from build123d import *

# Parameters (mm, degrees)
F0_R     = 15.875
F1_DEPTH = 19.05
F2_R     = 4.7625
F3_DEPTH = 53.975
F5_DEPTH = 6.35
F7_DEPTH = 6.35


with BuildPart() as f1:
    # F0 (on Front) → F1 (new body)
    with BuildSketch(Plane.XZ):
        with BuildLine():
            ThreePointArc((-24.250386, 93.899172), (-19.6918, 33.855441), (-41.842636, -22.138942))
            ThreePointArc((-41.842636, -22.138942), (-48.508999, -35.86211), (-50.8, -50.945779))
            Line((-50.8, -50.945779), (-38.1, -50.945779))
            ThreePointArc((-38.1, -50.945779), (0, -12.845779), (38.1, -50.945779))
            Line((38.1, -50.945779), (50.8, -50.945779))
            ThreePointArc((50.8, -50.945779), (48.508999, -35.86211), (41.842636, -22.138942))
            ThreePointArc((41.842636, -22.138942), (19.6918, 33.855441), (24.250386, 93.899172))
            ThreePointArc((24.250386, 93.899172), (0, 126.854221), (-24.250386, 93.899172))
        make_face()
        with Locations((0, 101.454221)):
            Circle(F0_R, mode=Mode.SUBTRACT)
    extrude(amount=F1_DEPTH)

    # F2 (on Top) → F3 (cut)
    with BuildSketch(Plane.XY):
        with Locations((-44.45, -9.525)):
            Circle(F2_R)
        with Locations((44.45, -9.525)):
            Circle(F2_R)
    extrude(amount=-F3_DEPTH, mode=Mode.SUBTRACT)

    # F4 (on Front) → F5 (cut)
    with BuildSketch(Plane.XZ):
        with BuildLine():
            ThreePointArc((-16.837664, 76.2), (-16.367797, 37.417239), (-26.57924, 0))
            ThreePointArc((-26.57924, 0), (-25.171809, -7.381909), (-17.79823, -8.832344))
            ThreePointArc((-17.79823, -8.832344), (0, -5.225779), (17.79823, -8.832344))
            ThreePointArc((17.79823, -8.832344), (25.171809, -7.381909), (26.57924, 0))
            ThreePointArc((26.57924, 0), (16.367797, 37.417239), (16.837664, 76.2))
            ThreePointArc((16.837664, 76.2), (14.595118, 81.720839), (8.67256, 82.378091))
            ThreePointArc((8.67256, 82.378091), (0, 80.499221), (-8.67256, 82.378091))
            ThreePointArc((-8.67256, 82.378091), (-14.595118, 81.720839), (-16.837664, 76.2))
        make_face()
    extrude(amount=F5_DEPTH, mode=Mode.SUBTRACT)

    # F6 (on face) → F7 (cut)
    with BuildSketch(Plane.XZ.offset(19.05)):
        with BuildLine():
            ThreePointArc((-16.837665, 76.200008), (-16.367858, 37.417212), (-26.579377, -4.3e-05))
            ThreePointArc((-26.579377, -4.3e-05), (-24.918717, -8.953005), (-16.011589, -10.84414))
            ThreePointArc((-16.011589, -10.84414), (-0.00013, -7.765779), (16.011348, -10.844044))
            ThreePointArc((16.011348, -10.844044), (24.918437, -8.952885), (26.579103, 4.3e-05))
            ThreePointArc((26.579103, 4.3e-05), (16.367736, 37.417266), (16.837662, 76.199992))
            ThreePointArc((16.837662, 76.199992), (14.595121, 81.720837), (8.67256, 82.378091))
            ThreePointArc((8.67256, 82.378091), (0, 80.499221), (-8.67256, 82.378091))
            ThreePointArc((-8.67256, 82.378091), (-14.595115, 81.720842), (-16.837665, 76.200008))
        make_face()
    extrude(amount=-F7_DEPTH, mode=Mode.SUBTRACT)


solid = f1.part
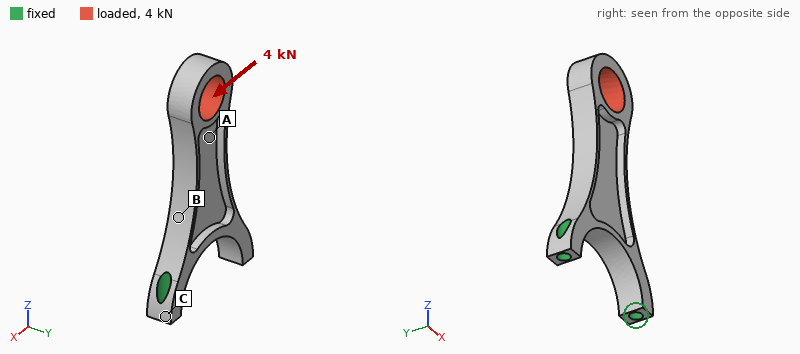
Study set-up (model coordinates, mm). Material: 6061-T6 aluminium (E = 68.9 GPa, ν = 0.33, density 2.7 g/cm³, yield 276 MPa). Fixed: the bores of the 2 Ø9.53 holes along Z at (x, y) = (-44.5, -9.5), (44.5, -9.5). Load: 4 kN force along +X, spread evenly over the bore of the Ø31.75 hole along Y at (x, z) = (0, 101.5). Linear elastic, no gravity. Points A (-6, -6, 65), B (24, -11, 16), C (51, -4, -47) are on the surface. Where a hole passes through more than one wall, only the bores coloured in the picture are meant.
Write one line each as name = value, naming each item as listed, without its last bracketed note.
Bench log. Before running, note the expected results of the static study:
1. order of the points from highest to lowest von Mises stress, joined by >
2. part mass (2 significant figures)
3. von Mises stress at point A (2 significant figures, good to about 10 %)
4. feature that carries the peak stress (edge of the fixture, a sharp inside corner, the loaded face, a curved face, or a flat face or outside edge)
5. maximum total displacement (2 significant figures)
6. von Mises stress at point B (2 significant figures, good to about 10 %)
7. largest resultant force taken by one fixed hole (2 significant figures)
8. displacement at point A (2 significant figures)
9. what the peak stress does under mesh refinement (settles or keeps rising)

order of the points from highest to lowest von Mises stress, joined by > = B > A > C
part mass = 220 g
von Mises stress at point A = 45 MPa
feature that carries the peak stress = edge of the fixture
maximum total displacement = 0.62 mm
von Mises stress at point B = 100 MPa
largest resultant force taken by one fixed hole = 7.5 kN
displacement at point A = 0.22 mm
what the peak stress does under mesh refinement = keeps rising
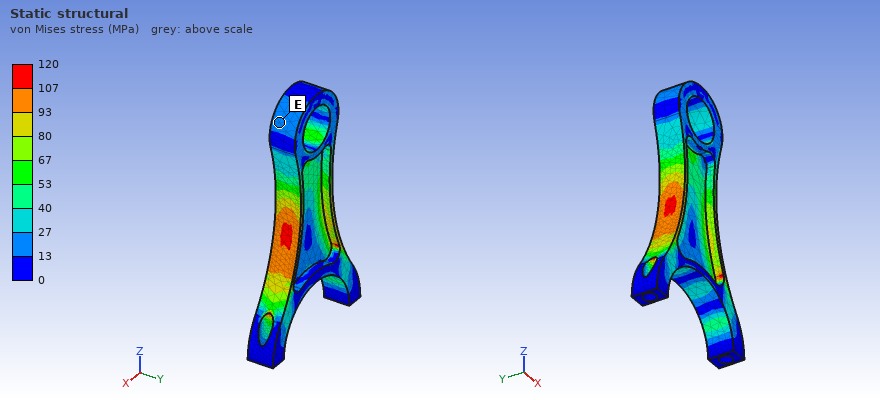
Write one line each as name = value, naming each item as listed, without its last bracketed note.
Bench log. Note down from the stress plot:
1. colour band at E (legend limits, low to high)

colour band at E = 13 to 27 MPa
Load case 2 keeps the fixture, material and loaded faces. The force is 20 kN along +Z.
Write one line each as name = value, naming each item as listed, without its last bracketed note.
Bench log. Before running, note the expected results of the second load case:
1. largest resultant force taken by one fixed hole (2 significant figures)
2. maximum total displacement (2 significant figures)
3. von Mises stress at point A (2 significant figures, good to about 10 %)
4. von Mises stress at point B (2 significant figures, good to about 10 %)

largest resultant force taken by one fixed hole = 12 kN
maximum total displacement = 0.16 mm
von Mises stress at point A = 50 MPa
von Mises stress at point B = 72 MPa
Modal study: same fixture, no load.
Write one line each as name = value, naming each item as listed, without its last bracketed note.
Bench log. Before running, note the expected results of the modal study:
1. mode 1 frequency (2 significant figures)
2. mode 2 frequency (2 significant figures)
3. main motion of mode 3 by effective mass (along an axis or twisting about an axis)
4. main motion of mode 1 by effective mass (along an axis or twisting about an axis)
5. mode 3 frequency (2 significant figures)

mode 1 frequency = 400 Hz
mode 2 frequency = 1300 Hz
main motion of mode 3 by effective mass = along X
main motion of mode 1 by effective mass = along Y
mode 3 frequency = 1700 Hz
